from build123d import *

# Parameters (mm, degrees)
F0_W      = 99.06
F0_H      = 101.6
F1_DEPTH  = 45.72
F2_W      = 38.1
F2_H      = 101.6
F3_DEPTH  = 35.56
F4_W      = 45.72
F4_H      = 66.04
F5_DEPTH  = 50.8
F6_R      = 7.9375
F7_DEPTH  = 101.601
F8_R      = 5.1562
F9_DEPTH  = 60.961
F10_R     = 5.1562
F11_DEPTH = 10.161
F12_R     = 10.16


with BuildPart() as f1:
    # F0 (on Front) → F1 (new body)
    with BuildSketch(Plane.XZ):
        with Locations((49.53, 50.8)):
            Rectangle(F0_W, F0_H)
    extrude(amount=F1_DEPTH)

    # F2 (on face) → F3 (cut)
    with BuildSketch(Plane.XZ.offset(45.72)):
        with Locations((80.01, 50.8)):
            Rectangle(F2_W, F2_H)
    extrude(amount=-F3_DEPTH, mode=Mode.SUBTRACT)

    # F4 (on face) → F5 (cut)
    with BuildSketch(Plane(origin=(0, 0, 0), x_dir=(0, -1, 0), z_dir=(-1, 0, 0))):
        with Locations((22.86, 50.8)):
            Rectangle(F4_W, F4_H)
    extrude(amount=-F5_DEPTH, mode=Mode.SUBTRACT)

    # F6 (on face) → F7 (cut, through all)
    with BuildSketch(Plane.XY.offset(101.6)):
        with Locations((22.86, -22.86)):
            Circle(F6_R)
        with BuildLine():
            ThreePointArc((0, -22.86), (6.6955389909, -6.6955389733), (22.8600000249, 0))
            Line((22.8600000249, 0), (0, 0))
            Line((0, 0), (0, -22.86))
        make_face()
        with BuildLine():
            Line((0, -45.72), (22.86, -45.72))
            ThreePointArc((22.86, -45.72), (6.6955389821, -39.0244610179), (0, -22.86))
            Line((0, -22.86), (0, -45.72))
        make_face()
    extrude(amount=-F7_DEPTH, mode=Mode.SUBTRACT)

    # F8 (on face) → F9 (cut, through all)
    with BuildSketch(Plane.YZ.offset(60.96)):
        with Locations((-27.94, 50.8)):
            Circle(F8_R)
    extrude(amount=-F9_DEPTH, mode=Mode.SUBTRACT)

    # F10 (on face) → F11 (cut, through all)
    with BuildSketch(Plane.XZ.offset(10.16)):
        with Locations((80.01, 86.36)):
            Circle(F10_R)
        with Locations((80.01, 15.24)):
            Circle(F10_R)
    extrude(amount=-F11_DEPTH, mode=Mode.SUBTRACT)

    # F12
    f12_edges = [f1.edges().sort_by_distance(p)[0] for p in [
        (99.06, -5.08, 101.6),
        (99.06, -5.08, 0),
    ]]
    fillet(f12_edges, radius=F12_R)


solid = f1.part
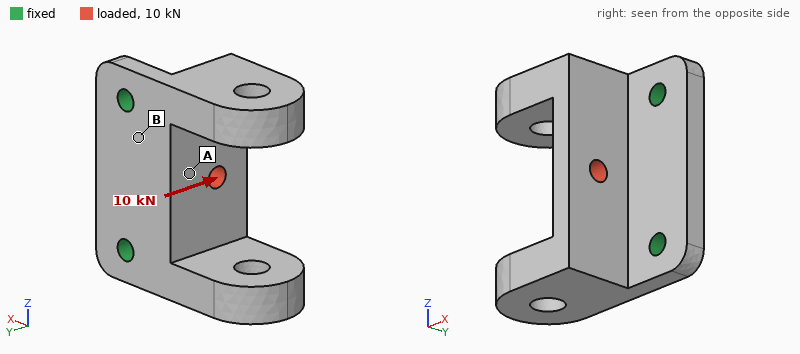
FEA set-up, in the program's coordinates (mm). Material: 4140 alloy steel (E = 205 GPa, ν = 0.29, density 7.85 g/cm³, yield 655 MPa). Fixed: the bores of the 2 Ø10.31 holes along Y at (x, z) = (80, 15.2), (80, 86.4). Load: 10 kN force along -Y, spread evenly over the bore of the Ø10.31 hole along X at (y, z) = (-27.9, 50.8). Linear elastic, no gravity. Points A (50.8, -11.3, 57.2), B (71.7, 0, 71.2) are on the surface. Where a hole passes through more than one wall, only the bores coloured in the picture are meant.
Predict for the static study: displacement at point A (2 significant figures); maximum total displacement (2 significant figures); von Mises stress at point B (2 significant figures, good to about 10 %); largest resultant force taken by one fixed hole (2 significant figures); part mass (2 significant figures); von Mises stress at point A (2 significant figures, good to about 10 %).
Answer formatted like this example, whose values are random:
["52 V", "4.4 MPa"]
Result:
["0.048 mm", "0.14 mm", "58 MPa", "5.1 kN", "1.2 kg", "22 MPa"]
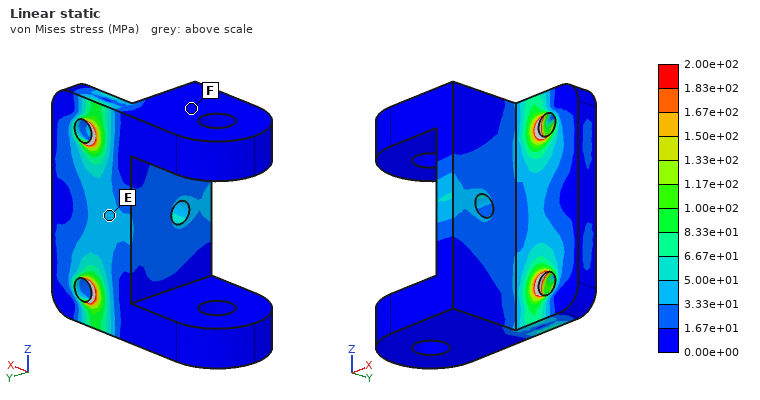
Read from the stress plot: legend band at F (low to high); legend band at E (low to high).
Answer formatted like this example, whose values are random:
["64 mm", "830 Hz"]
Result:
["0.00e+00 to 1.67e+01 MPa", "3.33e+01 to 5.00e+01 MPa"]
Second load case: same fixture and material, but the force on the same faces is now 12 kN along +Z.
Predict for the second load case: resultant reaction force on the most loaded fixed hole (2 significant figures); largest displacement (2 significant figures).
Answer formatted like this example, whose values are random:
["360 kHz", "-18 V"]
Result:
["7.8 kN", "47 µm"]
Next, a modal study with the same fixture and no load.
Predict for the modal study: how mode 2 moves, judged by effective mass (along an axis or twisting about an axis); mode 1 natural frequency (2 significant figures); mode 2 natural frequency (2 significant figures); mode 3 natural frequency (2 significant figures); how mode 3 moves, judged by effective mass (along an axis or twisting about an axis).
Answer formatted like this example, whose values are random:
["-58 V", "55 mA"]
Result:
["twisting about X", "1100 Hz", "1500 Hz", "2900 Hz", "along Z"]
